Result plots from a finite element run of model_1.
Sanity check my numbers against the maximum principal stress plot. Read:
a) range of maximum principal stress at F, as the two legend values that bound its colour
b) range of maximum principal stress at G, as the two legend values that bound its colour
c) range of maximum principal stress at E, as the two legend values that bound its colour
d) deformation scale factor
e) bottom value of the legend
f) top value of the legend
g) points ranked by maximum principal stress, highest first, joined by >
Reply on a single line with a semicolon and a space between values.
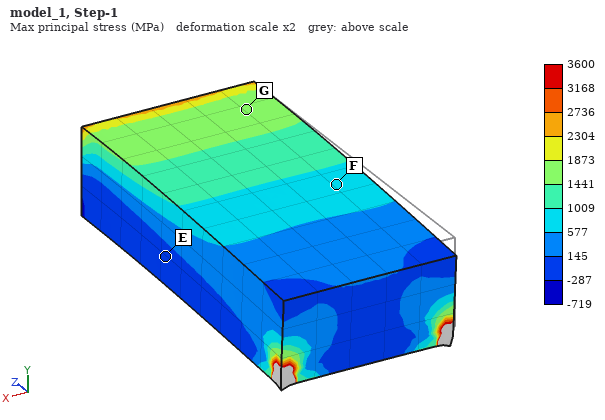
577 to 1009 MPa; 1441 to 1873 MPa; -287 to 145 MPa; 2; -719 MPa; 3600 MPa; G > F > E
